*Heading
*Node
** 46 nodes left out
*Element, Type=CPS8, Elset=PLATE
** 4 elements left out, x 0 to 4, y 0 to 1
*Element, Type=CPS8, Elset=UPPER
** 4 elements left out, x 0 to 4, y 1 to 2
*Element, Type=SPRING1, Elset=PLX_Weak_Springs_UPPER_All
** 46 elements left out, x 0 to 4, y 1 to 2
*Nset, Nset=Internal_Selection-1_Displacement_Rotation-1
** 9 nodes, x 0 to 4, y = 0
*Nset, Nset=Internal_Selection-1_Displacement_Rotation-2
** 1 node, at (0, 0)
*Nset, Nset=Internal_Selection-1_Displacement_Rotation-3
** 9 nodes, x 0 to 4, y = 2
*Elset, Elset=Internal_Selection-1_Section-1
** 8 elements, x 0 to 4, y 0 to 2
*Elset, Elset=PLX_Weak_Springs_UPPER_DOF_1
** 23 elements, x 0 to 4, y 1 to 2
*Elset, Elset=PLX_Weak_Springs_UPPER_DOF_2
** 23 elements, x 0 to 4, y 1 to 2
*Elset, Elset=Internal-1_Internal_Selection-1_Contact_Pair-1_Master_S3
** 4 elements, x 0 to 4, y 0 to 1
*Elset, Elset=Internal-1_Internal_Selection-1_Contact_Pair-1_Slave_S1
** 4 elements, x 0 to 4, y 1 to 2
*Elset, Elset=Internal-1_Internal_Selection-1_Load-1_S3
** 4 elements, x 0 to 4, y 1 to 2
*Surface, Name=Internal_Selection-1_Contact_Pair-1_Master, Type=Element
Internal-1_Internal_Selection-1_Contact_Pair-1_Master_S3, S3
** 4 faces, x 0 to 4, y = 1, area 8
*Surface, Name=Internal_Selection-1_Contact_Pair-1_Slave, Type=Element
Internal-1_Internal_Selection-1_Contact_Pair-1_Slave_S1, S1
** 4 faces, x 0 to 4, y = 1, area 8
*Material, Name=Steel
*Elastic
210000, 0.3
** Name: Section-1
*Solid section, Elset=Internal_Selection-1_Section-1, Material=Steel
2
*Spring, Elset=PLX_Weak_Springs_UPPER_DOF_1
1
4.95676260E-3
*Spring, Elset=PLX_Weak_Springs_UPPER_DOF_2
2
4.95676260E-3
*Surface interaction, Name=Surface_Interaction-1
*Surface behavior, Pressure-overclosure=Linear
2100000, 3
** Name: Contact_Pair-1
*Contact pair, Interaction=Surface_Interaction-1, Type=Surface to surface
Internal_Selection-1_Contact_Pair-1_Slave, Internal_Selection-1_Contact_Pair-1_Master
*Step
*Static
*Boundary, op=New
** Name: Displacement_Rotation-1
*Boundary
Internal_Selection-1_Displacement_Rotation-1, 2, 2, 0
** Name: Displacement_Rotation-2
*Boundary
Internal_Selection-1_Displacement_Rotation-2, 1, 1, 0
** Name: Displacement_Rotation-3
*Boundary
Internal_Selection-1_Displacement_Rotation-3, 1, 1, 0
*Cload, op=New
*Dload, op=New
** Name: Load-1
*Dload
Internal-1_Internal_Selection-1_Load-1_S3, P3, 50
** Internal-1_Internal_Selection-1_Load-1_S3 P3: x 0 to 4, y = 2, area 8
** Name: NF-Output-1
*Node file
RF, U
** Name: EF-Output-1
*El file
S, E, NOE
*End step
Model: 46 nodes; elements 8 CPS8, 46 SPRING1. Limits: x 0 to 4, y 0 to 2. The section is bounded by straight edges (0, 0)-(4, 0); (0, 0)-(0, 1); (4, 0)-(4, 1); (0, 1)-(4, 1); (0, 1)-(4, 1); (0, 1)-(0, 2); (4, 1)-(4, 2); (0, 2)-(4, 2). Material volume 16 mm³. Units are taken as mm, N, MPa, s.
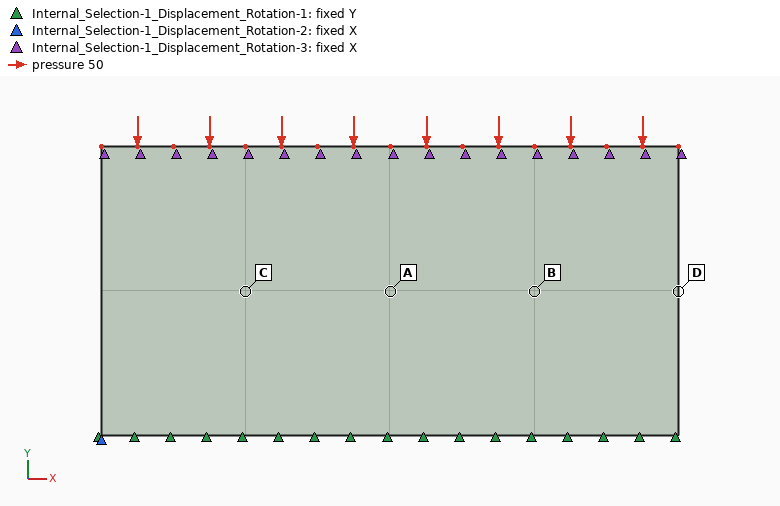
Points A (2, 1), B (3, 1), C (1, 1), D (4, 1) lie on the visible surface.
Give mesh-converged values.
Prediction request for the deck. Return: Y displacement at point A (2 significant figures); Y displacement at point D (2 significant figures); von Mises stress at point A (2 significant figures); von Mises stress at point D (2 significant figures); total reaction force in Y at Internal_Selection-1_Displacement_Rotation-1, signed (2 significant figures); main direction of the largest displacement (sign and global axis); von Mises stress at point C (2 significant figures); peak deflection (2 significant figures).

-2.8e-04 mm
-2.0e-04 mm
51 MPa
42 MPa
400 N
-Y
52 MPa
5.1e-04 mm
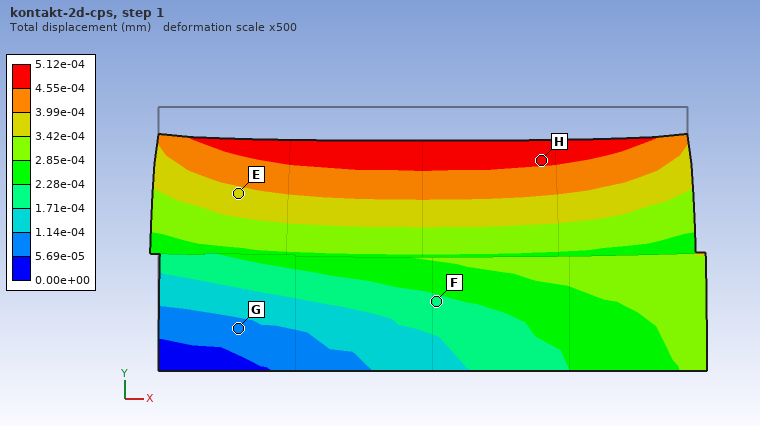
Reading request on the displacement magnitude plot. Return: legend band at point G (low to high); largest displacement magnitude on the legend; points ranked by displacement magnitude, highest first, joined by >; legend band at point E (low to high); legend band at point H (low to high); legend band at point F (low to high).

5.69e-05 to 1.14e-04 mm
5.12e-04 mm
H > E > F > G
3.42e-04 to 3.99e-04 mm
4.55e-04 to 5.12e-04 mm
1.71e-04 to 2.28e-04 mm
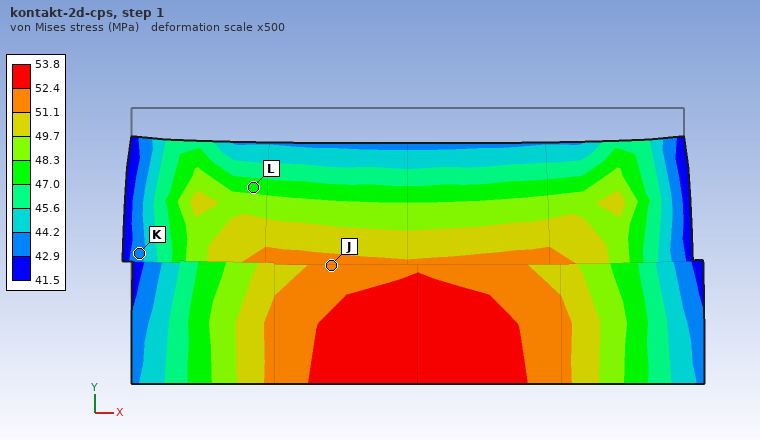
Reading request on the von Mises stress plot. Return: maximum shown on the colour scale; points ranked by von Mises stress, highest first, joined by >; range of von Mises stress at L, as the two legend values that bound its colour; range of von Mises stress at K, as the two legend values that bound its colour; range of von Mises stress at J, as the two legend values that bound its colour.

53.8 MPa
J > L > K
47.0 to 48.3 MPa
42.9 to 44.2 MPa
51.1 to 52.4 MPa
